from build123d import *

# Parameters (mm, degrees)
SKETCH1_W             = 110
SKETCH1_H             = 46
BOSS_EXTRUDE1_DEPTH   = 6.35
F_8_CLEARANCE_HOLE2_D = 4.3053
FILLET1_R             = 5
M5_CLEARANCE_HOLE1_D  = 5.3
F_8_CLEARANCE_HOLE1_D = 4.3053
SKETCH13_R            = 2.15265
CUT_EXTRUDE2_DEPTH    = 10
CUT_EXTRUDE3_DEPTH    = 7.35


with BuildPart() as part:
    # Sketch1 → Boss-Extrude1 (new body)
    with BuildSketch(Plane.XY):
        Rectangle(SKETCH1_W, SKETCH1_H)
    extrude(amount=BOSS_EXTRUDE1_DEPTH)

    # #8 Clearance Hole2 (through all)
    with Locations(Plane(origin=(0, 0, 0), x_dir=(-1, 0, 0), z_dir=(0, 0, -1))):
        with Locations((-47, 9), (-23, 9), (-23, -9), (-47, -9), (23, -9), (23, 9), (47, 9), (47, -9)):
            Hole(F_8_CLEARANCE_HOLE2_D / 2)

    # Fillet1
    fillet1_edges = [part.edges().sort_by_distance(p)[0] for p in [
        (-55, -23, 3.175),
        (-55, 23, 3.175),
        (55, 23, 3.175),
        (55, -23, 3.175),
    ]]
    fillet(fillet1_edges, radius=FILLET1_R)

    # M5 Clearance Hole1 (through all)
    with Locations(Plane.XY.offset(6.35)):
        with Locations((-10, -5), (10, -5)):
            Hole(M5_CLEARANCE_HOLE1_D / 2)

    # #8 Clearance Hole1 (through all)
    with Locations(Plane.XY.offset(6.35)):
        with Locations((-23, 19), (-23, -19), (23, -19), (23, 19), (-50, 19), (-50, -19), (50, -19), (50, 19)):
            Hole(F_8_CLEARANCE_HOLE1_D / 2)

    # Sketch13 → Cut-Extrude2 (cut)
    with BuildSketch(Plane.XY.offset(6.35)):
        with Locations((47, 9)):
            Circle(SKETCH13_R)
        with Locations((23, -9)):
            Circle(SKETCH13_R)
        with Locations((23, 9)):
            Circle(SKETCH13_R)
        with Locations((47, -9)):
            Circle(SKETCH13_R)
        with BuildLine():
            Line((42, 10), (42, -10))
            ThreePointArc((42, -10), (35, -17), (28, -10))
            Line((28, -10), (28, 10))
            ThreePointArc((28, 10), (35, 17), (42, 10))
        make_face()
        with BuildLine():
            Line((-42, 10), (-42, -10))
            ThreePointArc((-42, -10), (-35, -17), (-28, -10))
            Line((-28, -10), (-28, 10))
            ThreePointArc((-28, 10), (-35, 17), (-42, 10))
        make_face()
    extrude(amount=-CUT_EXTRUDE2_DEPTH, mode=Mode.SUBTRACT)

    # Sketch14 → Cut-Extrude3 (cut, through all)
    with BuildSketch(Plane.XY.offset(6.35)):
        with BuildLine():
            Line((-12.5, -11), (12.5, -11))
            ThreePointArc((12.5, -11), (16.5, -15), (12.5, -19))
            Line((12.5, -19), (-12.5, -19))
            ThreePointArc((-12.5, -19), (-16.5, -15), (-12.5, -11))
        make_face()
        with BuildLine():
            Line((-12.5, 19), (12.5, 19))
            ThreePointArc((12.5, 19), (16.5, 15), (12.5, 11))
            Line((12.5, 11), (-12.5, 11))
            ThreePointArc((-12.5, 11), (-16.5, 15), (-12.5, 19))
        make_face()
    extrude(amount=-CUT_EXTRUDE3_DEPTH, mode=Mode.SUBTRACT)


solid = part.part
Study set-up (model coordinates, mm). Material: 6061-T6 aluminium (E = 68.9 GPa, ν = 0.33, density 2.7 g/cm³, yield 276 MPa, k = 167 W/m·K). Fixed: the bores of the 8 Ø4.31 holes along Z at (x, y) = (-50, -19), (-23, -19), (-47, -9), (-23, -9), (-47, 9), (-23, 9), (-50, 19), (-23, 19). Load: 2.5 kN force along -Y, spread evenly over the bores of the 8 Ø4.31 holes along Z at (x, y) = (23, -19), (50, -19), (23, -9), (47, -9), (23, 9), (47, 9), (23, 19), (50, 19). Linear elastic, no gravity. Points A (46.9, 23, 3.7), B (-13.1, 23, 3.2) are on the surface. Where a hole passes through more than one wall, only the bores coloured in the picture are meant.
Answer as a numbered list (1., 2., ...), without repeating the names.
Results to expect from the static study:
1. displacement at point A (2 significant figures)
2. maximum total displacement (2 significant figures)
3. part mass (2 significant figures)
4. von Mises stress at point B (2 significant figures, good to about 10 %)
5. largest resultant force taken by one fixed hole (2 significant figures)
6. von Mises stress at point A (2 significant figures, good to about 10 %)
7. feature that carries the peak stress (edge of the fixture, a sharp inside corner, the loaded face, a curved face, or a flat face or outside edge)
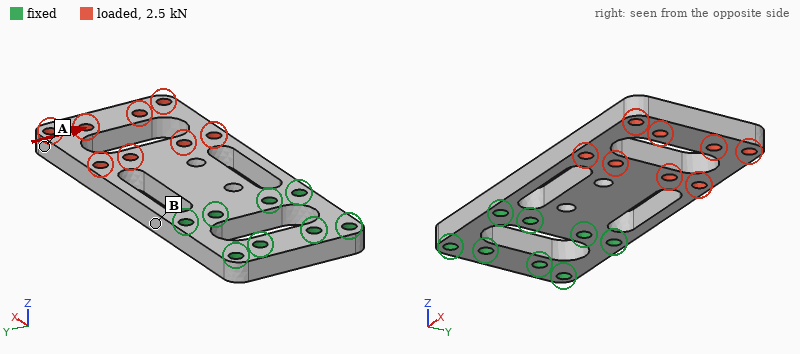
1. 0.21 mm
2. 0.22 mm
3. 58 g
4. 97 MPa
5. 2.6 kN
6. 24 MPa
7. a curved face
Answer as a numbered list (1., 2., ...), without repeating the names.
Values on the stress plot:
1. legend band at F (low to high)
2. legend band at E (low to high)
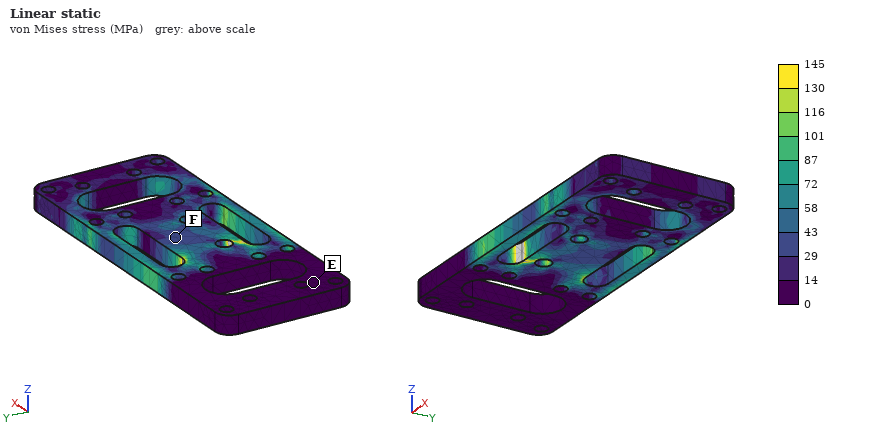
1. 29 to 43 MPa
2. 0 to 14 MPa
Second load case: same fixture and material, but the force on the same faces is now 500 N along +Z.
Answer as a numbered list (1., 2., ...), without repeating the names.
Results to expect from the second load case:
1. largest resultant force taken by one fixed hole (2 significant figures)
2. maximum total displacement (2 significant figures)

1. 260 N
2. 1.2 mm
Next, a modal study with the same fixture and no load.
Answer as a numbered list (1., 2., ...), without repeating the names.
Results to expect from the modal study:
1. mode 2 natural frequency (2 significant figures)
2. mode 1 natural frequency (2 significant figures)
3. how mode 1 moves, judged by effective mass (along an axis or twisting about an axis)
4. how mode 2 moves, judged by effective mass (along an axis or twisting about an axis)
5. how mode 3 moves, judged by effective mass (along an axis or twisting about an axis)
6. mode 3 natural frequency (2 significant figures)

1. 2500 Hz
2. 820 Hz
3. along Z
4. twisting about X
5. along Y
6. 4000 Hz
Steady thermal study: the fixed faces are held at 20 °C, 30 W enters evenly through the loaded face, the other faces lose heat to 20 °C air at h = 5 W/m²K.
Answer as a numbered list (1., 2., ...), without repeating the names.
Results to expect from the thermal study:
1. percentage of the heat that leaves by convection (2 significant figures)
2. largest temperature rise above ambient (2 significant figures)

1. 4.6 %
2. 68 K
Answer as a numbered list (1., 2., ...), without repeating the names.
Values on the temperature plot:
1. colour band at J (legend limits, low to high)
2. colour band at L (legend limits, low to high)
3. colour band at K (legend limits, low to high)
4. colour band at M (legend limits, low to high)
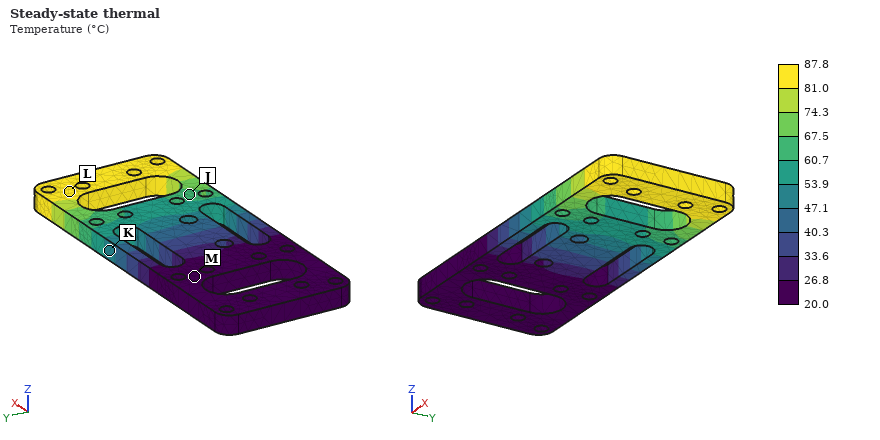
1. 60.7 to 67.5 °C
2. 81.0 to 87.8 °C
3. 47.1 to 53.9 °C
4. 20.0 to 26.8 °C
